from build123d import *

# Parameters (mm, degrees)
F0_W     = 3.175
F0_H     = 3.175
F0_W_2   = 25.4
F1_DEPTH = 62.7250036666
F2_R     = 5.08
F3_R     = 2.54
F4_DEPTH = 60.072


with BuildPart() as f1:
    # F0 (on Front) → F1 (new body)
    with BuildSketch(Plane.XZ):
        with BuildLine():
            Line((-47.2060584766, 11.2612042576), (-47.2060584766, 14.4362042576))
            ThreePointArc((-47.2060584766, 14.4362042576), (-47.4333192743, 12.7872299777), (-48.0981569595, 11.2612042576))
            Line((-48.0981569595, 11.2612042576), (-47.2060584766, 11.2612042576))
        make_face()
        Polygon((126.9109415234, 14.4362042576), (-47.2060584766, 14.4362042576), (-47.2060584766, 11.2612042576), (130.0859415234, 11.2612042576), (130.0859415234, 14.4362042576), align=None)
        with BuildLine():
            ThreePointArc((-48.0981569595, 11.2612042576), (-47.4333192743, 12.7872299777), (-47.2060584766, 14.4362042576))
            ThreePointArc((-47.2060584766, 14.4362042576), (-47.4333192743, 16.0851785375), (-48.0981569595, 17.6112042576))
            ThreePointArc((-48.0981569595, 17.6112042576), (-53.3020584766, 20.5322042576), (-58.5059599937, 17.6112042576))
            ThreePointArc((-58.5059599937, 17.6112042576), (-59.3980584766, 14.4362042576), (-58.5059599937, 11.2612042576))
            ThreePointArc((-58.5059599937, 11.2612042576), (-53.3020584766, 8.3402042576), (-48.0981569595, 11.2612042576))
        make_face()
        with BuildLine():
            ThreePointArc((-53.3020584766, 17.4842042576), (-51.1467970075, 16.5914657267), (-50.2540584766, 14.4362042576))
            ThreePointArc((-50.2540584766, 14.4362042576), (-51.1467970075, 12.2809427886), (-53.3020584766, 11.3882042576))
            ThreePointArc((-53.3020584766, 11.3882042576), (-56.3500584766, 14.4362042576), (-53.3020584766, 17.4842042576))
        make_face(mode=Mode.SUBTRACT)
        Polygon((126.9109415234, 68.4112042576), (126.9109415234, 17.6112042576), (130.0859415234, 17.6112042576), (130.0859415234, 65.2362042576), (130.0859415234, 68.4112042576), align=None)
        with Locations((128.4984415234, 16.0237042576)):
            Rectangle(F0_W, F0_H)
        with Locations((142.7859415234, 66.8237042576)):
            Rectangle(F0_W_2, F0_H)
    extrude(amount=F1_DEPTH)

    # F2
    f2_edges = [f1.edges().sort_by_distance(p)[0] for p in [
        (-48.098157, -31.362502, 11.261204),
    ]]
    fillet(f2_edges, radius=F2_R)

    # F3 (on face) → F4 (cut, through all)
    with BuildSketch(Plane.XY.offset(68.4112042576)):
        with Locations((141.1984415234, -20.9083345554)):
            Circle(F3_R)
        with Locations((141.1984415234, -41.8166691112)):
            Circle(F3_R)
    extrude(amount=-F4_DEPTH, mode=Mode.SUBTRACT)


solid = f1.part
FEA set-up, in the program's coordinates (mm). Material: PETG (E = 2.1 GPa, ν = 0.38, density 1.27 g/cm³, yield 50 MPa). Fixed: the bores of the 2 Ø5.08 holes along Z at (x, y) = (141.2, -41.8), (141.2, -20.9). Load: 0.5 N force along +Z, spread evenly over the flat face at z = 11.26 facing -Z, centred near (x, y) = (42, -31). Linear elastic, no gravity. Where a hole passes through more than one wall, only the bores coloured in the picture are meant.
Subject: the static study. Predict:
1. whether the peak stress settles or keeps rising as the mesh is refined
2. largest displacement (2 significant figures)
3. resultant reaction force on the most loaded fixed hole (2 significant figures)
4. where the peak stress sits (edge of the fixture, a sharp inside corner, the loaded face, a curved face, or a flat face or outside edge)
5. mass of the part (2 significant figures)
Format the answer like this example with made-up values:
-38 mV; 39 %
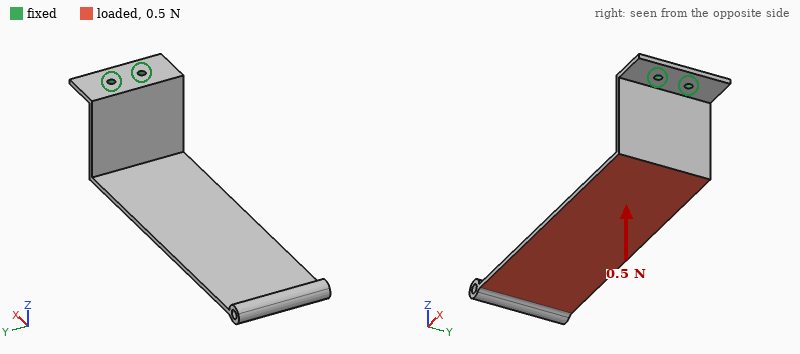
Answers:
keeps rising; 2.4 mm; 0.28 N; edge of the fixture; 72 g
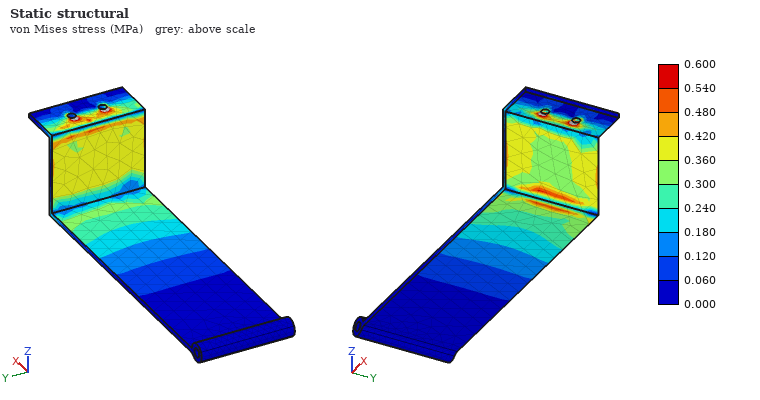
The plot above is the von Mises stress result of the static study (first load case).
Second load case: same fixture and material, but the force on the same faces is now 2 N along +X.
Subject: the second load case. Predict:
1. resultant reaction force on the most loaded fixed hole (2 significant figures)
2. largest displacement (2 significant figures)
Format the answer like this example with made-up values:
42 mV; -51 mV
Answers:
1.0 N; 2.3 mm
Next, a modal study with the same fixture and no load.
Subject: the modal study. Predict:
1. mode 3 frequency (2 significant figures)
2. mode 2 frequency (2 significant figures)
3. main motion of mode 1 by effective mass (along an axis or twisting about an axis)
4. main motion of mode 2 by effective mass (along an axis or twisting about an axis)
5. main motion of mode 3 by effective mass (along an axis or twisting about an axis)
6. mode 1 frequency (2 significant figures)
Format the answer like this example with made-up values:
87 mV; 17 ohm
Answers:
56 Hz; 23 Hz; along Z; along Y; along X; 11 Hz
